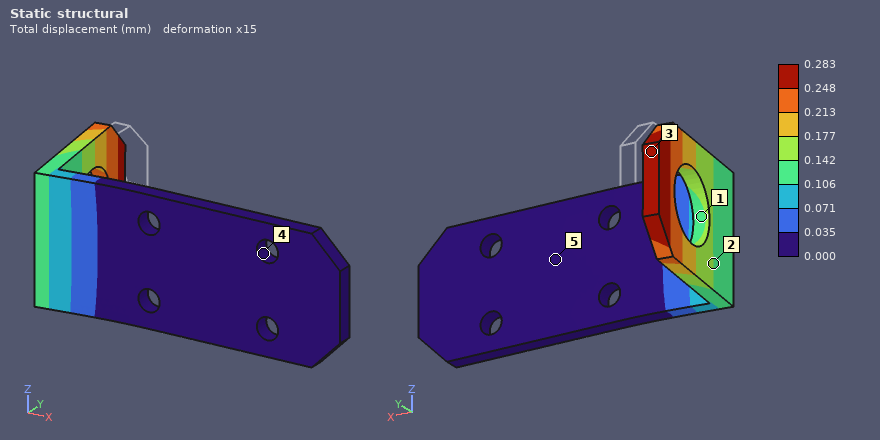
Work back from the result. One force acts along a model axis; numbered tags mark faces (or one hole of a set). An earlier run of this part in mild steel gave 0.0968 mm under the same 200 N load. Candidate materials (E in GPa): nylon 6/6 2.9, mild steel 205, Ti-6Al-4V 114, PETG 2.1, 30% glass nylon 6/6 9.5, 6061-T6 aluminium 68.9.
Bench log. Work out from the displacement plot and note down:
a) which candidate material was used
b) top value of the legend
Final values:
6061-T6 aluminium
0.283 mm
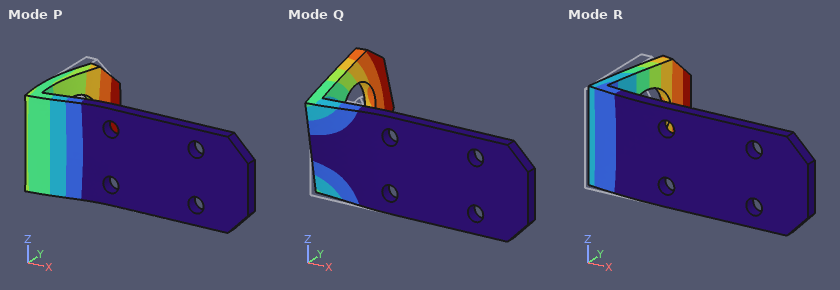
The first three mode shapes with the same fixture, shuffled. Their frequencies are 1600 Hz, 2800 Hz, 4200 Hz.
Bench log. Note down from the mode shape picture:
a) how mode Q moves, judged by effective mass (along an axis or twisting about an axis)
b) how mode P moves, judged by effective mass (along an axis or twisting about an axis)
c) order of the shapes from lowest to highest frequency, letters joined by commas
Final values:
along Z
along Y
R, Q, P
